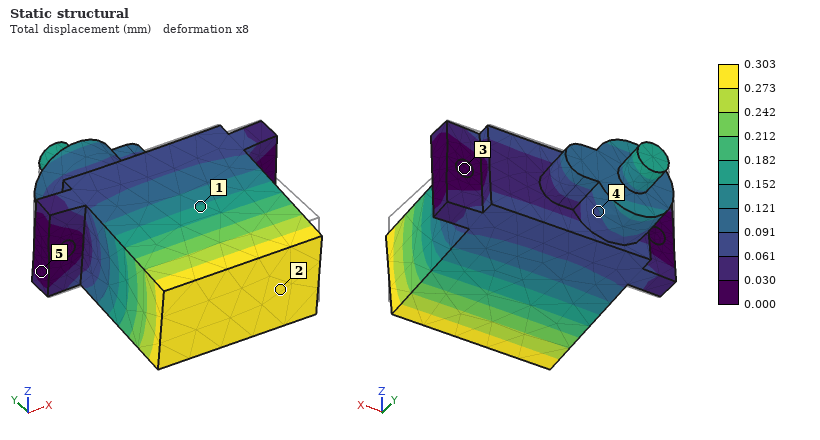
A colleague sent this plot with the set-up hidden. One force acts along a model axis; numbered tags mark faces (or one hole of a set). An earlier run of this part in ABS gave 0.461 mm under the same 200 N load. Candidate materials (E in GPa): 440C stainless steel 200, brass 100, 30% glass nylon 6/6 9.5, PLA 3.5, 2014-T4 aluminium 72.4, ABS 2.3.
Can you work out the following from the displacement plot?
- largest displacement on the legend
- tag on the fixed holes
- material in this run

0.303 mm
3
PLA
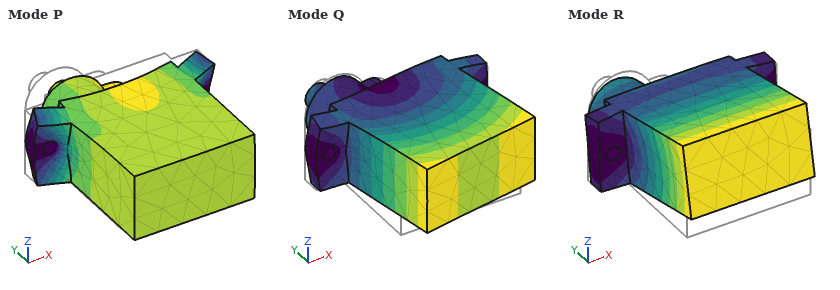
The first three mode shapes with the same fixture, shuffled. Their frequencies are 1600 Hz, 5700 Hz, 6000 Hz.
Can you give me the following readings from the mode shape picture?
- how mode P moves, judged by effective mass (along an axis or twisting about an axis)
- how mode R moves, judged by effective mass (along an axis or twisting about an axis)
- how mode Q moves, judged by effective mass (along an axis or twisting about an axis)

along Y
along Z
along X
